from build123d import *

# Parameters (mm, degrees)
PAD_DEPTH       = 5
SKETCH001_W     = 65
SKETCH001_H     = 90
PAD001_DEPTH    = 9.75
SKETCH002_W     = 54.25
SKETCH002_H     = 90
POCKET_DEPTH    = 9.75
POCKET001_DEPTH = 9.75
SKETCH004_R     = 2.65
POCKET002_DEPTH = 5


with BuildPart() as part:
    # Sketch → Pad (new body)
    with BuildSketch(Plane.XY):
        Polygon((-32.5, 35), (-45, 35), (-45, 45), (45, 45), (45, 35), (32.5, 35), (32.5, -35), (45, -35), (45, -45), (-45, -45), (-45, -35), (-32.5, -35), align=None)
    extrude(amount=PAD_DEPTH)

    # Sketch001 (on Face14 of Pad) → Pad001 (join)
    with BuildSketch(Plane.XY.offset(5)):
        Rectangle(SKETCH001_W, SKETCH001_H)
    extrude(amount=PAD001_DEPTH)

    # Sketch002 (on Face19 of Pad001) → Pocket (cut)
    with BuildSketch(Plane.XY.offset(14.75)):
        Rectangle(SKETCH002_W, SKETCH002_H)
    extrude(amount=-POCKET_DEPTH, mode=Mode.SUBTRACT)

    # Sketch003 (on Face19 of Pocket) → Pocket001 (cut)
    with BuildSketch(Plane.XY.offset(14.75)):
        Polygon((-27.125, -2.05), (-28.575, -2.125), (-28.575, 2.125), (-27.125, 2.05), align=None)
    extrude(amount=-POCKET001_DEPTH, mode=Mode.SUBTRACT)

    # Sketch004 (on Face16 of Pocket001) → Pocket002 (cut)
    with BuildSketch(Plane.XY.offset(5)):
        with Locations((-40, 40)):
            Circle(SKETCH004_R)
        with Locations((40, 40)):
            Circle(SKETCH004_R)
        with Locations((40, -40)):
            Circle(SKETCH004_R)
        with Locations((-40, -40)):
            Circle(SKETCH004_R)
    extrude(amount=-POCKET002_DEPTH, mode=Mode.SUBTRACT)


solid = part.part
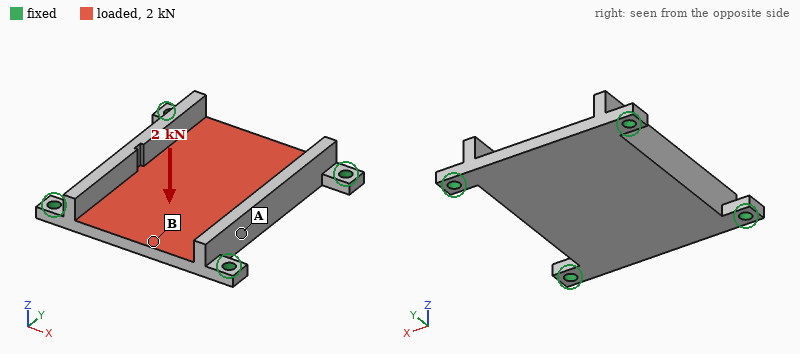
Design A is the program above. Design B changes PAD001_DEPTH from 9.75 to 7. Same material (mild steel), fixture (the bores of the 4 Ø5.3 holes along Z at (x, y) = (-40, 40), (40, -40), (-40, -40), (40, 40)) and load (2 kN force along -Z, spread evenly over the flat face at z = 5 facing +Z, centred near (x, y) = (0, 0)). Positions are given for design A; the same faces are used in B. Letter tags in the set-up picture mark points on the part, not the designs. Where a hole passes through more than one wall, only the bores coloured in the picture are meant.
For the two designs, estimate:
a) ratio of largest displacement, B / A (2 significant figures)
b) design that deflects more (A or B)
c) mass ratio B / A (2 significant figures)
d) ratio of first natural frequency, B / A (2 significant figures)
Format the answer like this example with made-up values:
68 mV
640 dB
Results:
1.1
B
0.94
0.97
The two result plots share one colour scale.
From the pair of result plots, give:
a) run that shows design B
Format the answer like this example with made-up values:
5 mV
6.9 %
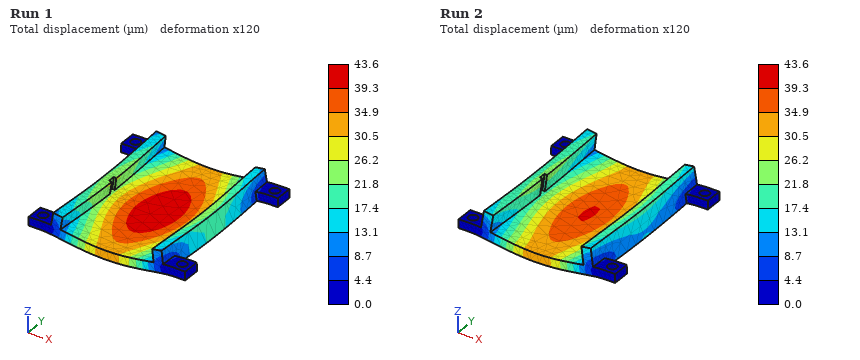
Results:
Run 1
